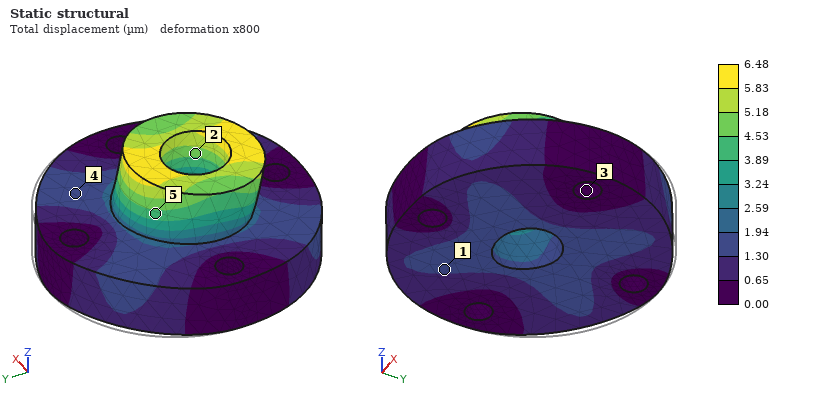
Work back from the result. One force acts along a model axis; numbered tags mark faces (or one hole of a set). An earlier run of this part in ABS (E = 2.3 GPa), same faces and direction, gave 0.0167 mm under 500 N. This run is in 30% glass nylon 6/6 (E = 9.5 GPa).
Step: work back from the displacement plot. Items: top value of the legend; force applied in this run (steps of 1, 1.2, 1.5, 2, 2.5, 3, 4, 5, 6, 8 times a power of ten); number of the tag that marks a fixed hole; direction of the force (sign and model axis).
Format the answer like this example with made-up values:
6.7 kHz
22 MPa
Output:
6.48 µm
800 N
3
-Y
